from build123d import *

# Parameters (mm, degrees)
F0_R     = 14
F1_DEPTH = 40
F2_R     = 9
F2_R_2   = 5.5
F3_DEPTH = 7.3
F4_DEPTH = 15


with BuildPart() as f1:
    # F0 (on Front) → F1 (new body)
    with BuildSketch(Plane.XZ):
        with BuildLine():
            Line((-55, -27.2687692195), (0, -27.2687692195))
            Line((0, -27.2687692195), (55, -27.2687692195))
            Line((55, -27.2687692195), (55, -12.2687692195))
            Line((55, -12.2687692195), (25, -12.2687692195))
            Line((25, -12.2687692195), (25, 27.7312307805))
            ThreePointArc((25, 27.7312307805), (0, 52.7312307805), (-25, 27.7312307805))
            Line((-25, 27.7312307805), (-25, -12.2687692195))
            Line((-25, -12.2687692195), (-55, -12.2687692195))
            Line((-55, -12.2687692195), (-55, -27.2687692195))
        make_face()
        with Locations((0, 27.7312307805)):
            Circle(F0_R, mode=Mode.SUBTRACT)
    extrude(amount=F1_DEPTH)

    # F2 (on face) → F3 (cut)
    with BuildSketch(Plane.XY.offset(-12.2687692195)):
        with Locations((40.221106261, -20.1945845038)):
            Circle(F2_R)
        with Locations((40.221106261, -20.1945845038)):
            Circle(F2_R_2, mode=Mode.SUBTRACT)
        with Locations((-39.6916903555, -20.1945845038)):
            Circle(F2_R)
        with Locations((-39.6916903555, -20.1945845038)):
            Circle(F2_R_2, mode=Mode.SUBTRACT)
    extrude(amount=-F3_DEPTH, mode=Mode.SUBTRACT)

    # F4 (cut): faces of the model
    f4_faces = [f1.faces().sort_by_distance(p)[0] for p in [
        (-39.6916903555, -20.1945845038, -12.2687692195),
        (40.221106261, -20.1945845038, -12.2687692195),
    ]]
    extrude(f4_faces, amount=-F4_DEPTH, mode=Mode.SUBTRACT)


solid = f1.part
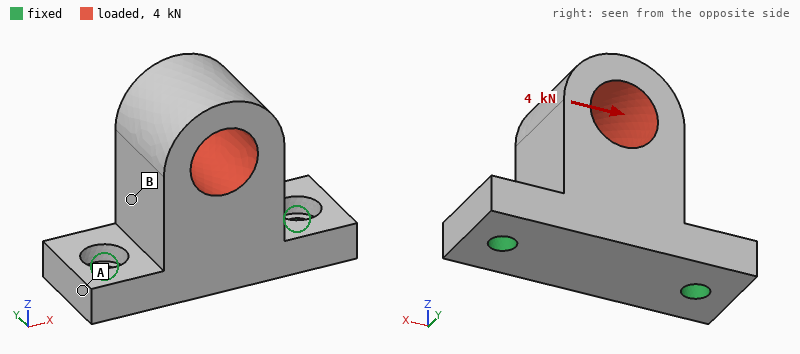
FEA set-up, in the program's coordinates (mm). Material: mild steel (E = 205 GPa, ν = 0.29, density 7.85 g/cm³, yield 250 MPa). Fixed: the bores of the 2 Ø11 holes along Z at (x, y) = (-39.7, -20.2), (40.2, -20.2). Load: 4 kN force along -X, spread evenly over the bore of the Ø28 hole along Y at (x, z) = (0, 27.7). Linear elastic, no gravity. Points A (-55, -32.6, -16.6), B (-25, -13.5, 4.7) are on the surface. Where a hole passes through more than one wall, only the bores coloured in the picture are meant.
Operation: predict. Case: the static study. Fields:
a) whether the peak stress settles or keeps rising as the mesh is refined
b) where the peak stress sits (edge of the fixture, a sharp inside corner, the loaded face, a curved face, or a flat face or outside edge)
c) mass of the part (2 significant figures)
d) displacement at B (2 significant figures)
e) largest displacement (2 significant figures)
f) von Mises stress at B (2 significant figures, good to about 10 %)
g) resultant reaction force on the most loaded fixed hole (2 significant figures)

keeps rising
edge of the fixture
1.2 kg
4.7 µm
13 µm
8.8 MPa
3.5 kN
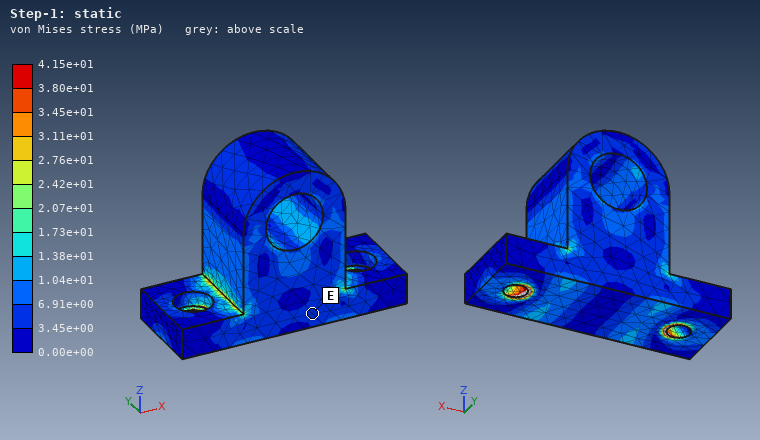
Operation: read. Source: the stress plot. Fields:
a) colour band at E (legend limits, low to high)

3.45e+00 to 6.91e+00 MPa
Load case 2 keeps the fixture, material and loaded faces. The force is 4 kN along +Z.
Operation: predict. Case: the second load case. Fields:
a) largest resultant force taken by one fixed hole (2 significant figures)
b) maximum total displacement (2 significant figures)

2.4 kN
3.7 µm
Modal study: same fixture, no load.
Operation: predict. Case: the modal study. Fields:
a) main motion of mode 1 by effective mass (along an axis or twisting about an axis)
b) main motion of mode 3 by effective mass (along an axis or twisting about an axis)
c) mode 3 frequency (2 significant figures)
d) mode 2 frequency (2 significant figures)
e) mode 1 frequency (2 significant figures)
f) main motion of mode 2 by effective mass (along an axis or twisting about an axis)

along Y
along Z
6100 Hz
4600 Hz
1600 Hz
along X
